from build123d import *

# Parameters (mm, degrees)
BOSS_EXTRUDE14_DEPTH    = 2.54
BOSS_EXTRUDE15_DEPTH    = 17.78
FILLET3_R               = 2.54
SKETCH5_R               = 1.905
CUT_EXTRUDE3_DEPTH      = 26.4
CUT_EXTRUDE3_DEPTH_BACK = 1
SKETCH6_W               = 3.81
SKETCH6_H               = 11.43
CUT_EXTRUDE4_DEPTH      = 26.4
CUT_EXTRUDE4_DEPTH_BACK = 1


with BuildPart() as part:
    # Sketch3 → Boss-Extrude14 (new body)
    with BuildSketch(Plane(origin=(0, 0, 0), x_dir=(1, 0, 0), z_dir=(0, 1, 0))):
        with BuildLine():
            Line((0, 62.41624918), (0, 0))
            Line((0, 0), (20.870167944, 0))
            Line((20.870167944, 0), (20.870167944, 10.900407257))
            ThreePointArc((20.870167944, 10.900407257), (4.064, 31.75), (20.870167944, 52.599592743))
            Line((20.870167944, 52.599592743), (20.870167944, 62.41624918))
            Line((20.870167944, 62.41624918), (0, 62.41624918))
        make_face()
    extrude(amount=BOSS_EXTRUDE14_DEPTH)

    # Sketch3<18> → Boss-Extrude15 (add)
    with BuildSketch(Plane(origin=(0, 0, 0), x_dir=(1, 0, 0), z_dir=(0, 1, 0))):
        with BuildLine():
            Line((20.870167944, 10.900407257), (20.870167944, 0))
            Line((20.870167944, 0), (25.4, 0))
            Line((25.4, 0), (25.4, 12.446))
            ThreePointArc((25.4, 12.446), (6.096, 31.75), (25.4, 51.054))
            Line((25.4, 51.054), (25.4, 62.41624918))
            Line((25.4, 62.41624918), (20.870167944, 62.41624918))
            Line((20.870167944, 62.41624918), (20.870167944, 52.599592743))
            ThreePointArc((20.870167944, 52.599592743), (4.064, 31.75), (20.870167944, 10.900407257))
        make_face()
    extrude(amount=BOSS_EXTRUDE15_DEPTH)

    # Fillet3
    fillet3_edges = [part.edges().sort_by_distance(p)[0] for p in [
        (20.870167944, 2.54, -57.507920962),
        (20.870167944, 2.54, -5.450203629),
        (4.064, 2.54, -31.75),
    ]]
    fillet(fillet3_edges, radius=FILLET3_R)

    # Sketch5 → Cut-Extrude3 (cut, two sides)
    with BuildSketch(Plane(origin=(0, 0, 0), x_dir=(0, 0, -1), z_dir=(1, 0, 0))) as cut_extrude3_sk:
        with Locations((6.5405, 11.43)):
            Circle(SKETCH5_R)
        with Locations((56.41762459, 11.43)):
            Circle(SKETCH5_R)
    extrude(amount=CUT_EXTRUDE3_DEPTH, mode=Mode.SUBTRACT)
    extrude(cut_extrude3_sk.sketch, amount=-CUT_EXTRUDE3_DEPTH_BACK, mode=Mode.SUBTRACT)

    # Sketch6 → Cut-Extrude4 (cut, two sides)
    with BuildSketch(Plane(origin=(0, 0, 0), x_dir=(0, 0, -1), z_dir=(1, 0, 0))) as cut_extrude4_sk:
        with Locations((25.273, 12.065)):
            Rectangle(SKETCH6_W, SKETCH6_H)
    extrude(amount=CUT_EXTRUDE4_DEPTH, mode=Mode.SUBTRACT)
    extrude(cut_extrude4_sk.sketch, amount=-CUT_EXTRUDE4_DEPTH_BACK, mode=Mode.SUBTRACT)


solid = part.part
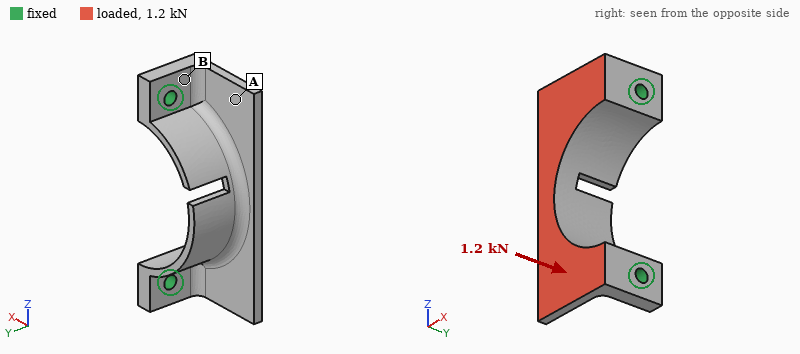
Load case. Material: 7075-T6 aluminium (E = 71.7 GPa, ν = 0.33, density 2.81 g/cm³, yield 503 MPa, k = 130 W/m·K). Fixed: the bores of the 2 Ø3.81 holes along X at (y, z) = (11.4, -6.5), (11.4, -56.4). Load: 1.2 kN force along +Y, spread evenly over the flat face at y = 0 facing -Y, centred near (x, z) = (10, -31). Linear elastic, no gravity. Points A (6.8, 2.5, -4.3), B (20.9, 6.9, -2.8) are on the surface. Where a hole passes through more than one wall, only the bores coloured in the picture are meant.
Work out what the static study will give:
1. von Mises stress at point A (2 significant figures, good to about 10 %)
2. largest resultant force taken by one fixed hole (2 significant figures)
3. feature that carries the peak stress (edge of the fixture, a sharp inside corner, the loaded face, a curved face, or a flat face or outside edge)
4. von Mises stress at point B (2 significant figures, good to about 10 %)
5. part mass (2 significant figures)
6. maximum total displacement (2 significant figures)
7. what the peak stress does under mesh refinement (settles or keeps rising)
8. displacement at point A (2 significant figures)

26 MPa
610 N
edge of the fixture
69 MPa
16 g
0.20 mm
keeps rising
0.12 mm
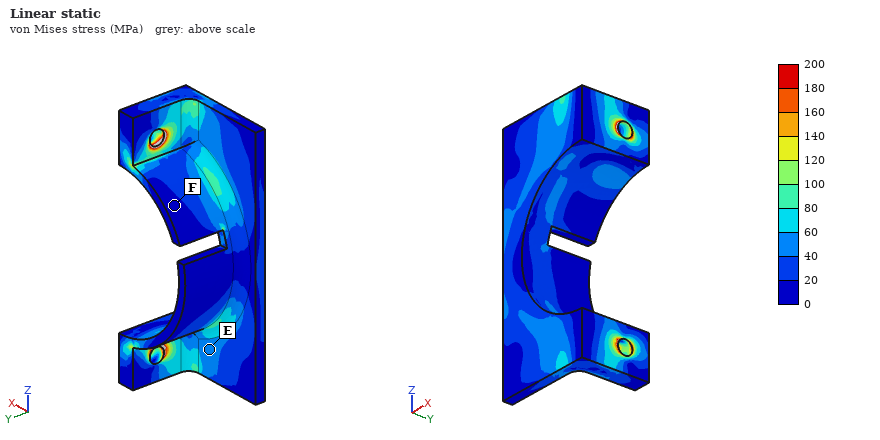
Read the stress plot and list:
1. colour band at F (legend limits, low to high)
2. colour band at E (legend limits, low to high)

0 to 20 MPa
40 to 60 MPa
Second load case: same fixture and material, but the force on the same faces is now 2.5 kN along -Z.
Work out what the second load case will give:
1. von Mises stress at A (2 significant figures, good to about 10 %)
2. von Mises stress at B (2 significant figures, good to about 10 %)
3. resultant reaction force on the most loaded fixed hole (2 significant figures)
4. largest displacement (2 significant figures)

25 MPa
74 MPa
1.4 kN
99 µm
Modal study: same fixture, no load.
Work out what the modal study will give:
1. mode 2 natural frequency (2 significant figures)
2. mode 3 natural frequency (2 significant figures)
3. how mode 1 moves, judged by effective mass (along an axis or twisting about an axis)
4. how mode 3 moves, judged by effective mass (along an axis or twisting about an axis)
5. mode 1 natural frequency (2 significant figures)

5900 Hz
8800 Hz
along Y
along Z
5400 Hz
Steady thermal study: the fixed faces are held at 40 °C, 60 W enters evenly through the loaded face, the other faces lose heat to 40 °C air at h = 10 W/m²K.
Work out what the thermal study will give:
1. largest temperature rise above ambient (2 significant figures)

65 K
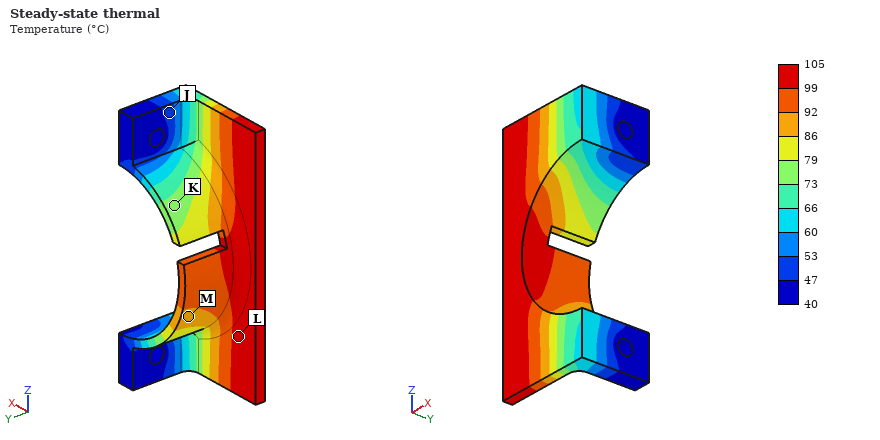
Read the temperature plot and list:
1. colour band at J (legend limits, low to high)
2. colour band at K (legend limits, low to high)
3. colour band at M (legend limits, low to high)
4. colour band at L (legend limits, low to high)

47 to 53 °C
73 to 79 °C
86 to 92 °C
99 to 105 °C
